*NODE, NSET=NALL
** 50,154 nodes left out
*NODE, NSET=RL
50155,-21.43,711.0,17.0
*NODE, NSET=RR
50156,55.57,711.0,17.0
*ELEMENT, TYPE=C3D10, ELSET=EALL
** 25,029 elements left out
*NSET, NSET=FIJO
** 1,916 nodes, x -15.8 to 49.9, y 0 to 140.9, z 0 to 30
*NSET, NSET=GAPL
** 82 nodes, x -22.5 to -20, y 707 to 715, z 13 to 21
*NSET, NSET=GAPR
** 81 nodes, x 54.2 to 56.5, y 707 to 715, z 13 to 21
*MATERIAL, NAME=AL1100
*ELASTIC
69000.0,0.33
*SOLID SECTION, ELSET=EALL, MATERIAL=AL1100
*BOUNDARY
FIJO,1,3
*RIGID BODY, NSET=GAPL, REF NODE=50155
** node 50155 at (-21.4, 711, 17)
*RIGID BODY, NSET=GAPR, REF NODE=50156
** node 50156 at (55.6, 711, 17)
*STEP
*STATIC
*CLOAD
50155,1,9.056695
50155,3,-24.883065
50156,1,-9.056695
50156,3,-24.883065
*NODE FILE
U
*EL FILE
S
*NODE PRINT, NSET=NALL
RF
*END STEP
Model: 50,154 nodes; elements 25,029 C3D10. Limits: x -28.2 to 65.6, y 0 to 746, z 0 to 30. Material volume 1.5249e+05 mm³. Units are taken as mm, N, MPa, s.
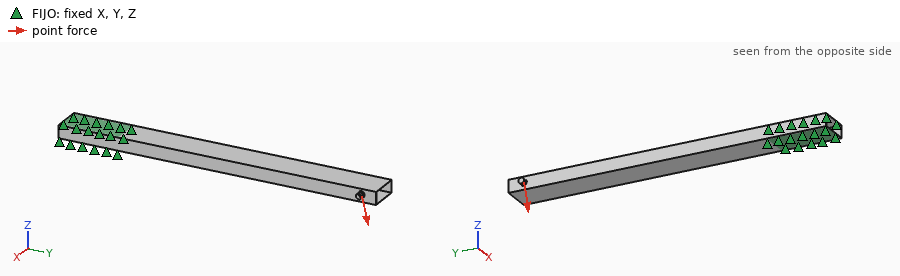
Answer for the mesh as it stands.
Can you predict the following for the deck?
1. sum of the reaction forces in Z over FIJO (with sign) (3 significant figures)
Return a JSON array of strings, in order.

["49.8 N"]
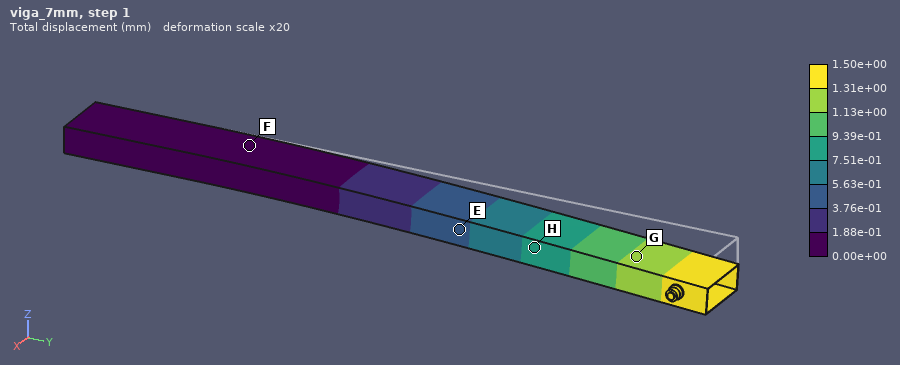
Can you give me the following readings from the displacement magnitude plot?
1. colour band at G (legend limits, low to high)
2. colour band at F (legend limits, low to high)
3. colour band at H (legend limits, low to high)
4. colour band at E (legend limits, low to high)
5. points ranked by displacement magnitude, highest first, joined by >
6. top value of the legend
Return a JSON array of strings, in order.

["1.13e+00 to 1.31e+00 mm", "0.00e+00 to 1.88e-01 mm", "7.51e-01 to 9.39e-01 mm", "3.76e-01 to 5.63e-01 mm", "G > H > E > F", "1.50e+00 mm"]
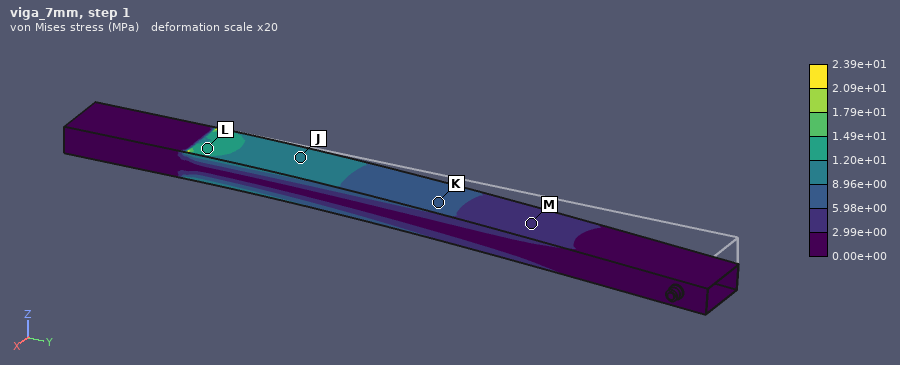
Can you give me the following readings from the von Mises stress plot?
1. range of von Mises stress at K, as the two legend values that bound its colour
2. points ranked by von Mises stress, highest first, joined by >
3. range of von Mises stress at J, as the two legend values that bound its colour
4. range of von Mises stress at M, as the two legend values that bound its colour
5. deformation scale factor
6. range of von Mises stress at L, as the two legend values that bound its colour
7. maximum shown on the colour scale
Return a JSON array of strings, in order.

["5.98e+00 to 8.96e+00 MPa", "L > J > K > M", "8.96e+00 to 1.20e+01 MPa", "2.99e+00 to 5.98e+00 MPa", "20", "1.20e+01 to 1.49e+01 MPa", "2.39e+01 MPa"]
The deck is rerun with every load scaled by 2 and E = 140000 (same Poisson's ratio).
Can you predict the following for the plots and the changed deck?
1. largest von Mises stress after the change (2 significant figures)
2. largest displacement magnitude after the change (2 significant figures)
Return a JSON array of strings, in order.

["48 MPa", "1.5 mm"]
